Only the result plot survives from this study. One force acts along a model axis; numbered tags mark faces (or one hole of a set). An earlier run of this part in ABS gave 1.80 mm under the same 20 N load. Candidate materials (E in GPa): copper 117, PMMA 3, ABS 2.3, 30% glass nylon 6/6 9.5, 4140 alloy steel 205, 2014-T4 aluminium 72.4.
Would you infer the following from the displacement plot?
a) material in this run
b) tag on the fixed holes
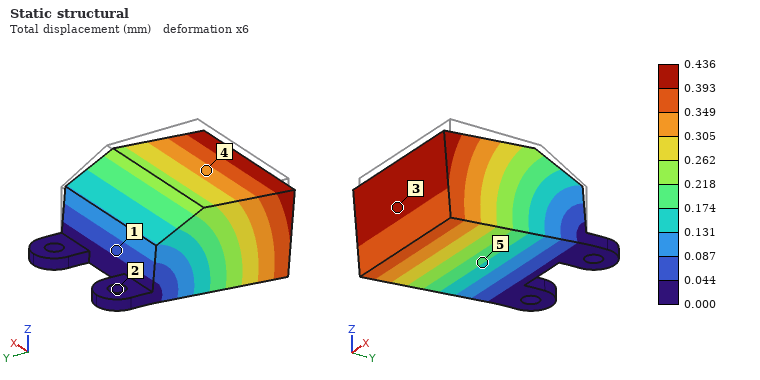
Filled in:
30% glass nylon 6/6
2
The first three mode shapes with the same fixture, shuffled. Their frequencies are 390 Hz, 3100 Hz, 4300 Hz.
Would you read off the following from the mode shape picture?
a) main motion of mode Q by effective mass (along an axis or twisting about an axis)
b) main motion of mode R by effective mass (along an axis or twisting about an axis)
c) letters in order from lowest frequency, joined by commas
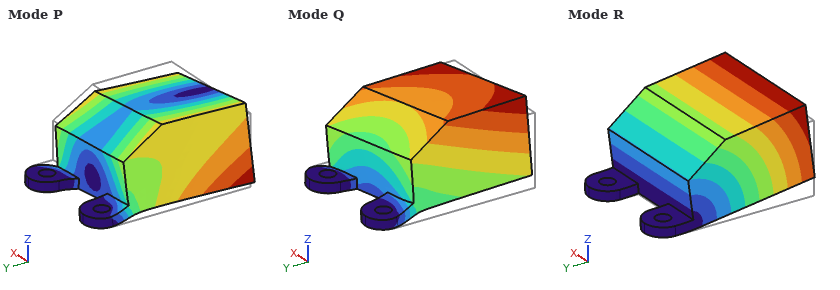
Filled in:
along X
along Z
R, Q, P
